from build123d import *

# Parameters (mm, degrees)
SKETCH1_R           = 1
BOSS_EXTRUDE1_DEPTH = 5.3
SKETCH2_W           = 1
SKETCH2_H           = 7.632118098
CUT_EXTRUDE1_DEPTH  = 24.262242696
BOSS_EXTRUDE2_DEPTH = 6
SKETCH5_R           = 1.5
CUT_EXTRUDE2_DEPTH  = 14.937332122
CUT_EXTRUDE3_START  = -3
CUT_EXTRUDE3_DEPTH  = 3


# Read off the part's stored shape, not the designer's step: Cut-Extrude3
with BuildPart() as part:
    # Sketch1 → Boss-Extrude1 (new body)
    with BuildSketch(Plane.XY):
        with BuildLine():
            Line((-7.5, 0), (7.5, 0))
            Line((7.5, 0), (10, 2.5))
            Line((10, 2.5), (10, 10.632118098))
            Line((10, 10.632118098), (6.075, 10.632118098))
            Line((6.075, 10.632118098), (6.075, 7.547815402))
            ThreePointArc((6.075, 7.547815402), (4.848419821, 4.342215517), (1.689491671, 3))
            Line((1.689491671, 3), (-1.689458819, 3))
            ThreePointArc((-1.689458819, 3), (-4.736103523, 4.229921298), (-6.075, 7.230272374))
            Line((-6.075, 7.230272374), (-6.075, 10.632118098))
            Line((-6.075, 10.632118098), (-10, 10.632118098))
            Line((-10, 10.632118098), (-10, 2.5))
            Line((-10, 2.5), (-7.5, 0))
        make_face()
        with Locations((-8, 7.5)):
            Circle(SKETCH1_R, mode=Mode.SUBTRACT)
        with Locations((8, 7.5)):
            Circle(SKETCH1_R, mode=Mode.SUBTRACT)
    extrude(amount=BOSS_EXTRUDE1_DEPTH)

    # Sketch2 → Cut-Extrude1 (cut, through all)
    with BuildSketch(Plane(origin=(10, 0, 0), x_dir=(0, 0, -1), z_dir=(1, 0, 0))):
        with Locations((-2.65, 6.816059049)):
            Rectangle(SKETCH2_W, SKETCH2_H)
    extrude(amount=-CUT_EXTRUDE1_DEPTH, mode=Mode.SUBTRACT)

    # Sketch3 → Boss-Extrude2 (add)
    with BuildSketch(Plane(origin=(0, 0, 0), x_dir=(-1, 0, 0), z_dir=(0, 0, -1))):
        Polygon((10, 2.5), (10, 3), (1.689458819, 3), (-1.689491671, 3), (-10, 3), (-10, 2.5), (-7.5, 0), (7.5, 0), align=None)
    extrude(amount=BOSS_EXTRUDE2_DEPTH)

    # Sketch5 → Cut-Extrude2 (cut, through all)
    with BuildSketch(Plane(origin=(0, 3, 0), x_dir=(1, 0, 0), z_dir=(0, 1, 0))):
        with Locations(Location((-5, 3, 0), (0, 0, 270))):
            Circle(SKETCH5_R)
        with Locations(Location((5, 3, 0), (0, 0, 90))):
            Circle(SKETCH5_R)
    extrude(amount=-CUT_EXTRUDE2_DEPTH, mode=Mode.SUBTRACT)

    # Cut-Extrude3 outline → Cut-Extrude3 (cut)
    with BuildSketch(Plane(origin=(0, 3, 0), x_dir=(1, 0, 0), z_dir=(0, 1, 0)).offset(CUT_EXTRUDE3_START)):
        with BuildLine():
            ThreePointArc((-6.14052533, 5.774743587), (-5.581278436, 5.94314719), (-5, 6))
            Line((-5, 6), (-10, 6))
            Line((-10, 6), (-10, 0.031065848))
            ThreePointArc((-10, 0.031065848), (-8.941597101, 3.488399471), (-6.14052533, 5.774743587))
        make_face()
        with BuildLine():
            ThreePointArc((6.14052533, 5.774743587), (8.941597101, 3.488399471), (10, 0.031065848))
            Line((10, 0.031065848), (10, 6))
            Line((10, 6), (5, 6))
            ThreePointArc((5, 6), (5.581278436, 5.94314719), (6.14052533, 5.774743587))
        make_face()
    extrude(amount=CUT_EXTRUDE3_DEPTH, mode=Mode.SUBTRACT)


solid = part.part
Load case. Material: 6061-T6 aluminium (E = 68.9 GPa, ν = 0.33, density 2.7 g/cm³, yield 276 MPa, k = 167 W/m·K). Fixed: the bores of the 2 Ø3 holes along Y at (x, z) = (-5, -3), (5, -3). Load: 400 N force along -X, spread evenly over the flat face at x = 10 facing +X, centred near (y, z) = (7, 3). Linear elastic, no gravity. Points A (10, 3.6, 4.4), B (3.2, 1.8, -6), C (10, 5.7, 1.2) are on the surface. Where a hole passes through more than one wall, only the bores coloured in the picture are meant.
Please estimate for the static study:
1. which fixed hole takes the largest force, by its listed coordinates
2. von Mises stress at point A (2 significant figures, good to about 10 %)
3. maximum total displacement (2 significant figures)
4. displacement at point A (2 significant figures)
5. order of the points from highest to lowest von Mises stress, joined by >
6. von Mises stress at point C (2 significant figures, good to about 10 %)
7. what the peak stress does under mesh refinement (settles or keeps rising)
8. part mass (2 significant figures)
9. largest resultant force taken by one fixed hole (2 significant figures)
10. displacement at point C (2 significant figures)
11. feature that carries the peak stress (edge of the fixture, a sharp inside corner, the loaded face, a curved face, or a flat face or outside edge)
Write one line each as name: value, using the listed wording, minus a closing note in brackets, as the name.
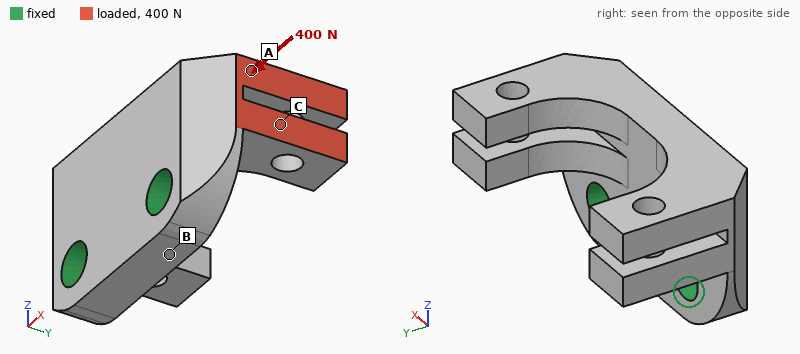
which fixed hole takes the largest force, by its listed coordinates: (5, -3)
von Mises stress at point A: 41 MPa
maximum total displacement: 65 µm
displacement at point A: 29 µm
order of the points from highest to lowest von Mises stress, joined by >: C > A > B
von Mises stress at point C: 74 MPa
what the peak stress does under mesh refinement: keeps rising
part mass: 2.2 g
largest resultant force taken by one fixed hole: 300 N
displacement at point C: 28 µm
feature that carries the peak stress: edge of the fixture
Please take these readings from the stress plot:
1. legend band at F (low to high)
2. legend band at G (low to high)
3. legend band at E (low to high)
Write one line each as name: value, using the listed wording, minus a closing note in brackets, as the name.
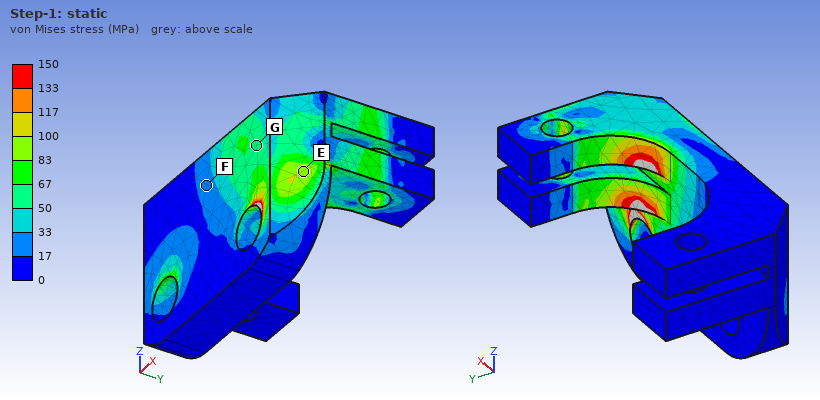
legend band at F: 17 to 33 MPa
legend band at G: 50 to 67 MPa
legend band at E: 83 to 100 MPa
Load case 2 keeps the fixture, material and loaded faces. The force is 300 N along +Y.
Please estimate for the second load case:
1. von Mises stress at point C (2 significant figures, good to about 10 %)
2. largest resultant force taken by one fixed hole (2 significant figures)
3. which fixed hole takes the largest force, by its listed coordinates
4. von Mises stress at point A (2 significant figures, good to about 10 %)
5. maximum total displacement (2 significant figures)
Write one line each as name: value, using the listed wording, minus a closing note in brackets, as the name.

von Mises stress at point C: 50 MPa
largest resultant force taken by one fixed hole: 360 N
which fixed hole takes the largest force, by its listed coordinates: (5, -3)
von Mises stress at point A: 33 MPa
maximum total displacement: 66 µm
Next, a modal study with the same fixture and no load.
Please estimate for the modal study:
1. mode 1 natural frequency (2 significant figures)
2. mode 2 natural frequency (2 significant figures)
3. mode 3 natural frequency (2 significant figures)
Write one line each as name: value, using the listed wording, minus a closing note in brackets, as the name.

mode 1 natural frequency: 17 kHz
mode 2 natural frequency: 18 kHz
mode 3 natural frequency: 24 kHz
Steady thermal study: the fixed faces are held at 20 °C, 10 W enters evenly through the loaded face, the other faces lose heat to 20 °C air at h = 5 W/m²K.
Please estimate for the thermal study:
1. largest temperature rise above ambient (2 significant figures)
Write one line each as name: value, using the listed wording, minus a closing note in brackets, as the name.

largest temperature rise above ambient: 31 K
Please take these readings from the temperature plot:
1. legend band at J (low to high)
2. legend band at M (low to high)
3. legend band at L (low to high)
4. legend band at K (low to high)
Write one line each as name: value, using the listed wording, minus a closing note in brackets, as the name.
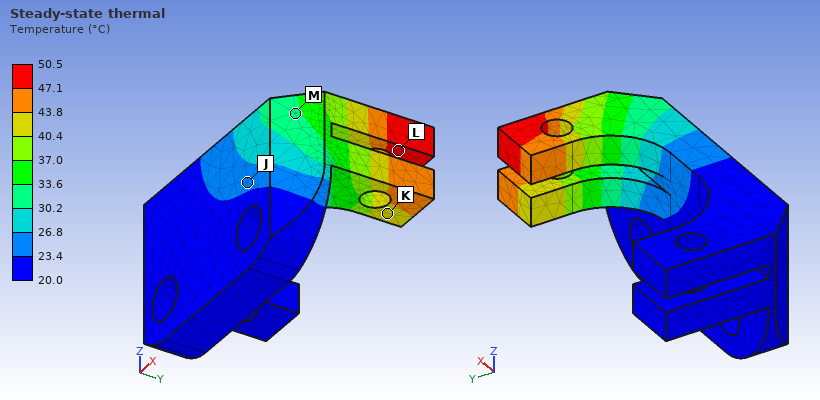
legend band at J: 23.4 to 26.8 °C
legend band at M: 30.2 to 33.6 °C
legend band at L: 47.1 to 50.5 °C
legend band at K: 40.4 to 43.8 °C
